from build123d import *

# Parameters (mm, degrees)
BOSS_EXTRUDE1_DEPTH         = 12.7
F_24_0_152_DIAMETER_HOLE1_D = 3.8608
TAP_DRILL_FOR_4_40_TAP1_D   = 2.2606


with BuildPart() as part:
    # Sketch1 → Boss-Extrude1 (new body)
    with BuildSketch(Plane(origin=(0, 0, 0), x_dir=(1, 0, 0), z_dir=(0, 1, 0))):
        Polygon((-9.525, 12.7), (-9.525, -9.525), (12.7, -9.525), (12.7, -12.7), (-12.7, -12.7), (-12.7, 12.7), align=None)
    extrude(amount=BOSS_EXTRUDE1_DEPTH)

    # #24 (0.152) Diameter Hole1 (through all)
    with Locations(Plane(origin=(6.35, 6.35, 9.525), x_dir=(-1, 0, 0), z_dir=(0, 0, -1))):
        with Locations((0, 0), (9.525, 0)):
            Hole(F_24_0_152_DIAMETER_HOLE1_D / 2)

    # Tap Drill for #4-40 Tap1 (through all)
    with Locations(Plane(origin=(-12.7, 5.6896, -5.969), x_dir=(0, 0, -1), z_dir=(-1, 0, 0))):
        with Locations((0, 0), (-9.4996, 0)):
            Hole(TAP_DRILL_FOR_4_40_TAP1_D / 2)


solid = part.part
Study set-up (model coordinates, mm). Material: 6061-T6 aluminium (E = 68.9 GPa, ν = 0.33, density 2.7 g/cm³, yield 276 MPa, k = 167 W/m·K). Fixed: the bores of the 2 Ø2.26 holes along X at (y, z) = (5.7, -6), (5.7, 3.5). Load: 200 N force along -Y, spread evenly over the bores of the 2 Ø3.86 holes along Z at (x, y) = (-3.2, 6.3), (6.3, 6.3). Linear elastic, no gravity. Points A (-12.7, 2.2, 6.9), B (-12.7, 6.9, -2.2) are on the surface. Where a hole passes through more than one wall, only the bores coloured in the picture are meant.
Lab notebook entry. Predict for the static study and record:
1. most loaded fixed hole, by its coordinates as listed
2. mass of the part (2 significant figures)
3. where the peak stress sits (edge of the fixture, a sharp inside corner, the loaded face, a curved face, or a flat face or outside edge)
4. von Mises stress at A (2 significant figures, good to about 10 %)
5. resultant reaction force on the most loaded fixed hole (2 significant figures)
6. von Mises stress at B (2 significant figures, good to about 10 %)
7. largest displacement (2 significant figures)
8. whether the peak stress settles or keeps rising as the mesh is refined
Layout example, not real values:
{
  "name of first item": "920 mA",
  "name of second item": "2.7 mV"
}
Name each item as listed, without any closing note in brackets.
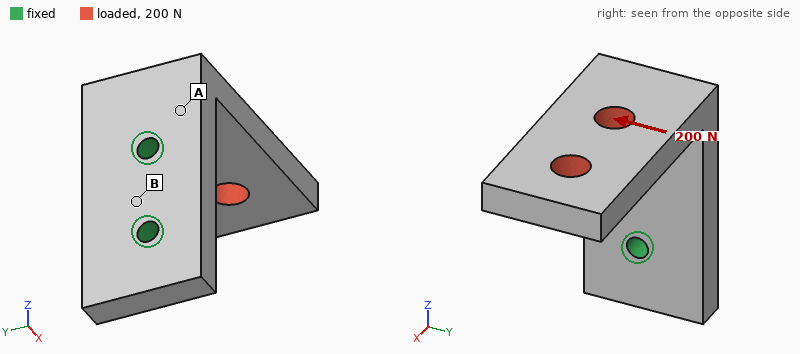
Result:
{
  "most loaded fixed hole, by its coordinates as listed": "(5.7, 3.5)",
  "mass of the part": "4.9 g",
  "where the peak stress sits": "edge of the fixture",
  "von Mises stress at A": "61 MPa",
  "resultant reaction force on the most loaded fixed hole": "310 N",
  "von Mises stress at B": "22 MPa",
  "largest displacement": "0.14 mm",
  "whether the peak stress settles or keeps rising as the mesh is refined": "keeps rising"
}
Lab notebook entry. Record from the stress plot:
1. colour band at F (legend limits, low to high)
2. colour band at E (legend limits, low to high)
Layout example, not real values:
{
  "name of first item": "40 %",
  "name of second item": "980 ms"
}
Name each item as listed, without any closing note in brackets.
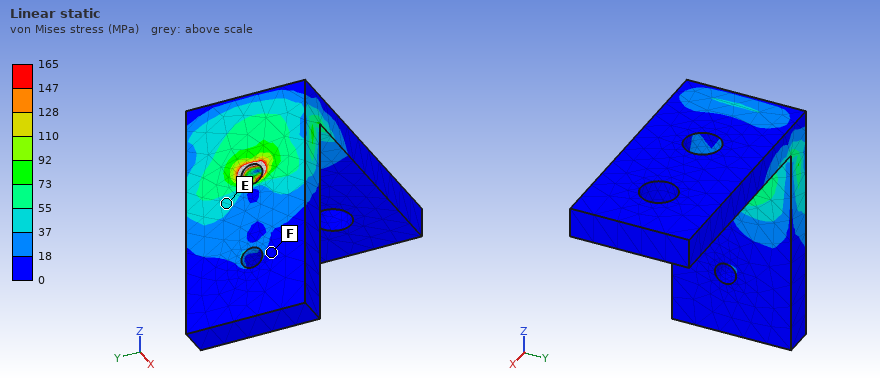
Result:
{
  "colour band at F": "0 to 18 MPa",
  "colour band at E": "37 to 55 MPa"
}
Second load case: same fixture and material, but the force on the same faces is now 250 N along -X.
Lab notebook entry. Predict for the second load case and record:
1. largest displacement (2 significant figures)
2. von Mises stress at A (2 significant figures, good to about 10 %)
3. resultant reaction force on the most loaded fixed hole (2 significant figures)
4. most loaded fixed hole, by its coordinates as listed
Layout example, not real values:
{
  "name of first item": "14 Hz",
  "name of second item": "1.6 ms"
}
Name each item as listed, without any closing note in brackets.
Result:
{
  "largest displacement": "84 µm",
  "von Mises stress at A": "42 MPa",
  "resultant reaction force on the most loaded fixed hole": "310 N",
  "most loaded fixed hole, by its coordinates as listed": "(5.7, 3.5)"
}
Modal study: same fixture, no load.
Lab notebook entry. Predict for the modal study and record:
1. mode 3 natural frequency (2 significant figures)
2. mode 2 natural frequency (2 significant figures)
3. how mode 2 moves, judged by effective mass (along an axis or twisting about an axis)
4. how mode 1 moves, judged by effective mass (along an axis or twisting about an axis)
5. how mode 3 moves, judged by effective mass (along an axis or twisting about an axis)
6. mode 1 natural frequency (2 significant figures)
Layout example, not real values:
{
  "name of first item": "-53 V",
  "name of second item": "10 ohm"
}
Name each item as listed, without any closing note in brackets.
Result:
{
  "mode 3 natural frequency": "13 kHz",
  "mode 2 natural frequency": "4700 Hz",
  "how mode 2 moves, judged by effective mass": "along Y",
  "how mode 1 moves, judged by effective mass": "along Z",
  "how mode 3 moves, judged by effective mass": "along X",
  "mode 1 natural frequency": "3100 Hz"
}
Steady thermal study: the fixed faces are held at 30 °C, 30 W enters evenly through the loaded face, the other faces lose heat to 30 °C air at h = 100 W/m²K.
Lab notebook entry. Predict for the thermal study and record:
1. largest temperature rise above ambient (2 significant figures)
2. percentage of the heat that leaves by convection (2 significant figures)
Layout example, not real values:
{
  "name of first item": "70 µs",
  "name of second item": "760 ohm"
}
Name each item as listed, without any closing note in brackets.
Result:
{
  "largest temperature rise above ambient": "83 K",
  "percentage of the heat that leaves by convection": "18 %"
}
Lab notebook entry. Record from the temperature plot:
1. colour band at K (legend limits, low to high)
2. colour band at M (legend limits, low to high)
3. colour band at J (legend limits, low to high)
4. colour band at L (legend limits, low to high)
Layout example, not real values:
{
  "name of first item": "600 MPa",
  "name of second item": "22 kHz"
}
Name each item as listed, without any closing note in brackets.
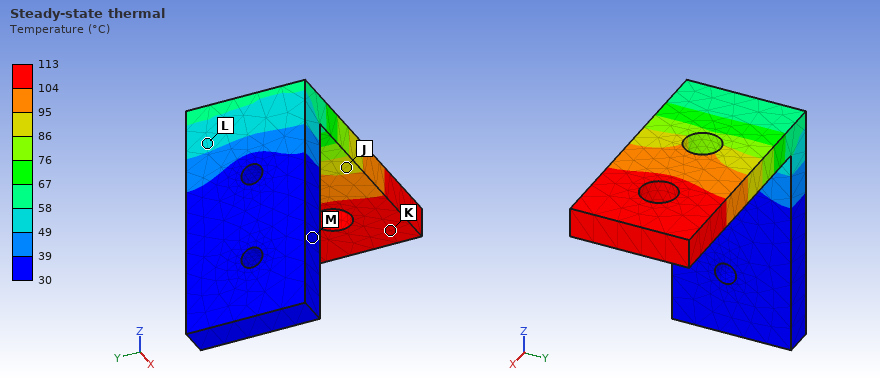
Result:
{
  "colour band at K": "104 to 113 °C",
  "colour band at M": "30 to 39 °C",
  "colour band at J": "86 to 95 °C",
  "colour band at L": "49 to 58 °C"
}
